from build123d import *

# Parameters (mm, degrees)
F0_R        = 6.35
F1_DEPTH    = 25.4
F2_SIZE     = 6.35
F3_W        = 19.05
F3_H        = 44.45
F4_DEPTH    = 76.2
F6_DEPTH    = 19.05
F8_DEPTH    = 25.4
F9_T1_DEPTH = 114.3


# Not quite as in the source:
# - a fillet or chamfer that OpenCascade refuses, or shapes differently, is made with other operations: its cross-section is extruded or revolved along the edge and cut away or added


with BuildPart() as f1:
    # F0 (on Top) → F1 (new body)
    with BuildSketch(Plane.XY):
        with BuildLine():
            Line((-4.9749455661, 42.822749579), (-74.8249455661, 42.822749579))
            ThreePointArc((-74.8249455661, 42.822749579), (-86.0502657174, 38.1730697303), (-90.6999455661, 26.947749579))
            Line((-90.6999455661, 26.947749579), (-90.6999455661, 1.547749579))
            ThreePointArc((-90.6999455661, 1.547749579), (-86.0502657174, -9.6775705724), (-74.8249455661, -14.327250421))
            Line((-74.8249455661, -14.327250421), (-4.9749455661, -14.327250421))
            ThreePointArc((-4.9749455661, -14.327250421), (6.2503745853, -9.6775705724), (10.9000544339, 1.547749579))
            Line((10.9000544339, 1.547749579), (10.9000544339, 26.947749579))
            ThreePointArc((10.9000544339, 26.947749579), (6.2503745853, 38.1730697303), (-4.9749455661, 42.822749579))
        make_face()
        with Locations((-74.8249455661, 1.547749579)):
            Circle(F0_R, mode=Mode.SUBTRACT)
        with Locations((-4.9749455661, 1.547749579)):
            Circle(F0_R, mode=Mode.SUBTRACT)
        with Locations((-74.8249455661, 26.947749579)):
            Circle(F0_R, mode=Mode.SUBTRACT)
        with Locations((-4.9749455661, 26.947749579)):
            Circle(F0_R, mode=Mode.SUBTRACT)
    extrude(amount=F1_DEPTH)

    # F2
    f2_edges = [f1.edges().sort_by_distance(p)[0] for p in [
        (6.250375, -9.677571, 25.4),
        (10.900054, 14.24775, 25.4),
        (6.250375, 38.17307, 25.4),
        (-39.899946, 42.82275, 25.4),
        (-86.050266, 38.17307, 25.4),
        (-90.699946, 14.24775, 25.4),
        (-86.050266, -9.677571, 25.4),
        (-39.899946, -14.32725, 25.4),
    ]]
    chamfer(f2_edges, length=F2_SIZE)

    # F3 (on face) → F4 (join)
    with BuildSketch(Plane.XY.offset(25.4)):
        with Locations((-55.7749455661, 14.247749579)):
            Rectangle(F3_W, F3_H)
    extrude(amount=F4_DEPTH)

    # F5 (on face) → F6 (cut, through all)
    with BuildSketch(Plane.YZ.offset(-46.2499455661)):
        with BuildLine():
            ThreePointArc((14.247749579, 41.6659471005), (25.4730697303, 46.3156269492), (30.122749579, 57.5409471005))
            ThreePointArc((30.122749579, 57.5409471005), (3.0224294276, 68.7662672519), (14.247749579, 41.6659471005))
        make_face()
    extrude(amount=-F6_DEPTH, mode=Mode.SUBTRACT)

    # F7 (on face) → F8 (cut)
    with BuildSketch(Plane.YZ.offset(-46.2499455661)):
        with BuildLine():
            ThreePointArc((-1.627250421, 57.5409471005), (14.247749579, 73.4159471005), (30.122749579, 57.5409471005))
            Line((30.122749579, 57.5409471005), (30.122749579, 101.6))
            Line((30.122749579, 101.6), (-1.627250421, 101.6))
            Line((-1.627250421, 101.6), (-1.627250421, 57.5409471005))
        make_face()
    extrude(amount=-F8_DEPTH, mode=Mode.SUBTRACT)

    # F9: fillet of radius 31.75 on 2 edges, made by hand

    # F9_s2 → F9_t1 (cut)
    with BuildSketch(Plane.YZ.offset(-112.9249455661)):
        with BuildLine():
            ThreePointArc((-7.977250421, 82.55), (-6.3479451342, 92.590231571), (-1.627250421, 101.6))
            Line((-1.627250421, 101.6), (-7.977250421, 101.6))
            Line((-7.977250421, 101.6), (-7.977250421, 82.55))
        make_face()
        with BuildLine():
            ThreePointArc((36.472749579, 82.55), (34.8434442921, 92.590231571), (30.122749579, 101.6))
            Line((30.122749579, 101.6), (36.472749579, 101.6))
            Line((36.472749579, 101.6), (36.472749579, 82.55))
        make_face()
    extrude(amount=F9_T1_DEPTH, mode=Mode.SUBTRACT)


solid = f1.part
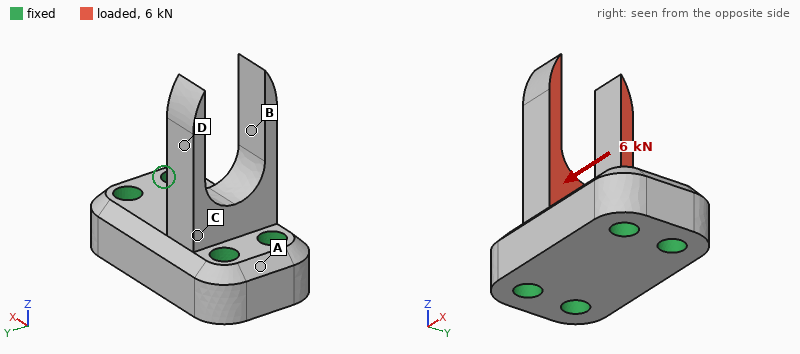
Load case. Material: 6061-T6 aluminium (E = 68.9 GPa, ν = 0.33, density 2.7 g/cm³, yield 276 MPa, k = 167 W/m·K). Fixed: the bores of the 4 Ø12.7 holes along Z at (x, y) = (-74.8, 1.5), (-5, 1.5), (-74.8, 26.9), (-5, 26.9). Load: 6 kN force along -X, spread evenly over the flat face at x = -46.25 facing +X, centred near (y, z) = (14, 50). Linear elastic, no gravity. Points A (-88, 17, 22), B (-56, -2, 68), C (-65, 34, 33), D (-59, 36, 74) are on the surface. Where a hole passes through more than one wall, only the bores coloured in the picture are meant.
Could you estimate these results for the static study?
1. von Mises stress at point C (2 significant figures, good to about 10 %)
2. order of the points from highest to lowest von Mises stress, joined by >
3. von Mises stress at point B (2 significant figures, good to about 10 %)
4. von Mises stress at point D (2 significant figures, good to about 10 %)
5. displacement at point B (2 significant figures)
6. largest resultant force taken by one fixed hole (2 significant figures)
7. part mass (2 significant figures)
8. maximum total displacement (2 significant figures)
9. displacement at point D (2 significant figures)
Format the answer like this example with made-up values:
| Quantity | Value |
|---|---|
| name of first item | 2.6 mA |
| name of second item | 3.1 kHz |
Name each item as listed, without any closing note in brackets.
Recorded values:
| Quantity | Value |
|---|---|
| von Mises stress at point C | 51 MPa |
| order of the points from highest to lowest von Mises stress, joined by > | C > B > D > A |
| von Mises stress at point B | 17 MPa |
| von Mises stress at point D | 9.9 MPa |
| displacement at point B | 0.11 mm |
| largest resultant force taken by one fixed hole | 2.9 kN |
| part mass | 410 g |
| maximum total displacement | 0.26 mm |
| displacement at point D | 0.13 mm |
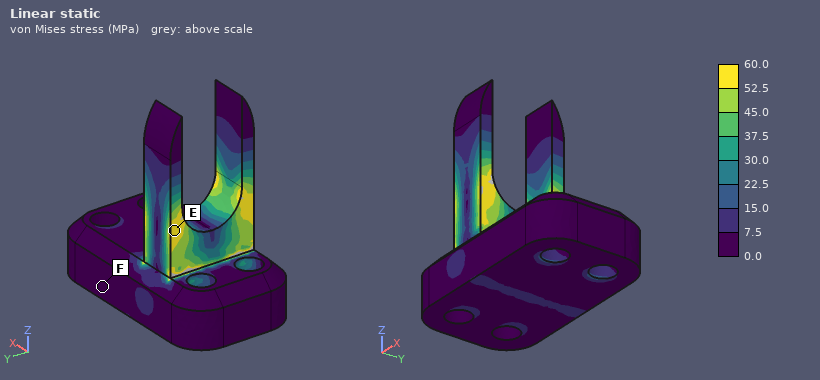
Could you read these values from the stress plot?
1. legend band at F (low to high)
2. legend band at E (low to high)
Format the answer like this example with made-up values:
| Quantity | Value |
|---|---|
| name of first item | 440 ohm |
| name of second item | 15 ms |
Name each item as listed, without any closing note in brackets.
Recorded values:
| Quantity | Value |
|---|---|
| legend band at F | 0.0 to 7.5 MPa |
| legend band at E | 52.5 to 60.0 MPa |
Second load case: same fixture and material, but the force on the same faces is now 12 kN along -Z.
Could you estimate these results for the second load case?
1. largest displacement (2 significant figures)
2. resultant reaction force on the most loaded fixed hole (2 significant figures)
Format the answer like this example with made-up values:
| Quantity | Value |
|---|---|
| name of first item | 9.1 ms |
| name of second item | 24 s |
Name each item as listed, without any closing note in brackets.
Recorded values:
| Quantity | Value |
|---|---|
| largest displacement | 0.23 mm |
| resultant reaction force on the most loaded fixed hole | 3.8 kN |
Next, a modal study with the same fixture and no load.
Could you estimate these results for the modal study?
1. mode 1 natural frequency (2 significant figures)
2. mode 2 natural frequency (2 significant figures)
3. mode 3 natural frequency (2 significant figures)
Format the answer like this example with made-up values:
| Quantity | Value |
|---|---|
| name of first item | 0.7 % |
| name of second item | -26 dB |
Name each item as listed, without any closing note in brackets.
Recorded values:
| Quantity | Value |
|---|---|
| mode 1 natural frequency | 2200 Hz |
| mode 2 natural frequency | 2200 Hz |
| mode 3 natural frequency | 3700 Hz |
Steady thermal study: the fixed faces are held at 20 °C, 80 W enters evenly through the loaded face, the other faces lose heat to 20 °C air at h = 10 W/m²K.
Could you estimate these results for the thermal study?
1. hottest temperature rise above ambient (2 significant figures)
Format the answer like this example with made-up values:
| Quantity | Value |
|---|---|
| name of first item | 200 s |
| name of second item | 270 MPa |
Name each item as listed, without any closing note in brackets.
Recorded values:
| Quantity | Value |
|---|---|
| hottest temperature rise above ambient | 36 K |
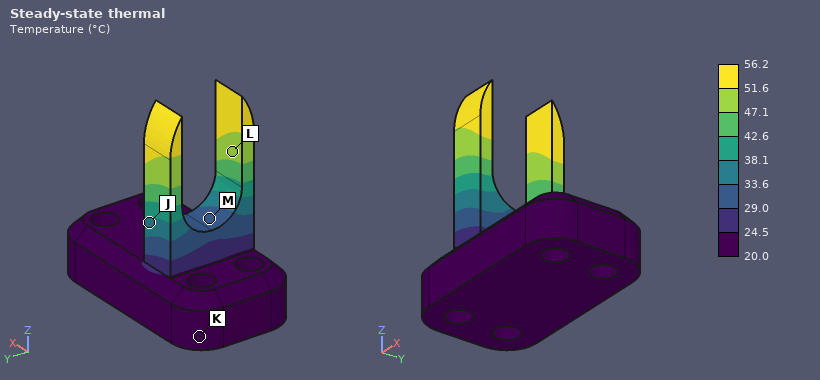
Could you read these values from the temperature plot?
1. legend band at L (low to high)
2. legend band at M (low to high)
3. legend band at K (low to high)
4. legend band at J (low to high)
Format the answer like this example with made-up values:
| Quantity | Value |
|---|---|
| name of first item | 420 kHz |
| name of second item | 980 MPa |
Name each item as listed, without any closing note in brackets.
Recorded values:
| Quantity | Value |
|---|---|
| legend band at L | 47.1 to 51.6 °C |
| legend band at M | 29.0 to 33.6 °C |
| legend band at K | 20.0 to 24.5 °C |
| legend band at J | 33.6 to 38.1 °C |
